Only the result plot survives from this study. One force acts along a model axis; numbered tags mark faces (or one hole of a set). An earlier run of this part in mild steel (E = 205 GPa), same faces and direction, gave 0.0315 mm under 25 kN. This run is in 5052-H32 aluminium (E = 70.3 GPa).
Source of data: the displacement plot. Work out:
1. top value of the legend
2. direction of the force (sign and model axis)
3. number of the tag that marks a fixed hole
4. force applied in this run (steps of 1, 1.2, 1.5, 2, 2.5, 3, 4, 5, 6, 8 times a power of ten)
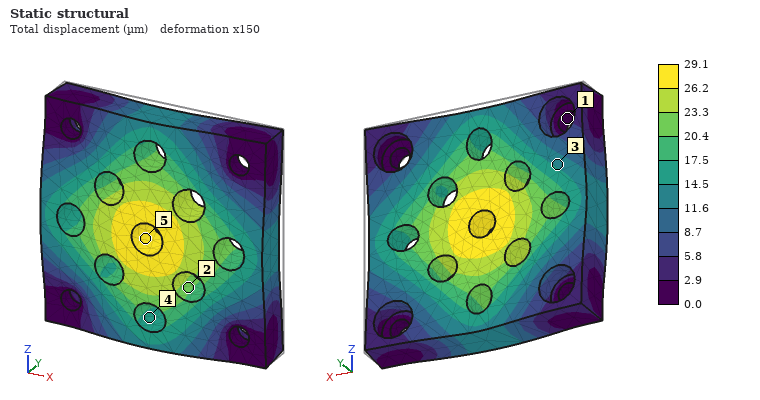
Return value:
29.1 µm
-Y
1
8 kN
